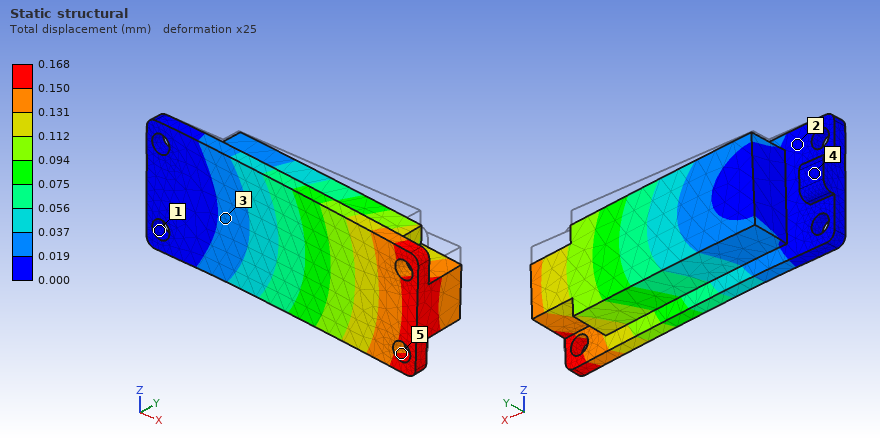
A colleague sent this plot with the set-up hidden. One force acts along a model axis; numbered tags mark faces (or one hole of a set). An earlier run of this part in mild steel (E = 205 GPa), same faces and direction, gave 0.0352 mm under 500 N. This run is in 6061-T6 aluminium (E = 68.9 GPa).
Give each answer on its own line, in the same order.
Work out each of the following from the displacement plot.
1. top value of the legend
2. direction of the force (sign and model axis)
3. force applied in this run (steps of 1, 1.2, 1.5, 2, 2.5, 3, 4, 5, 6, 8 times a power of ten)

0.168 mm
-Z
800 N
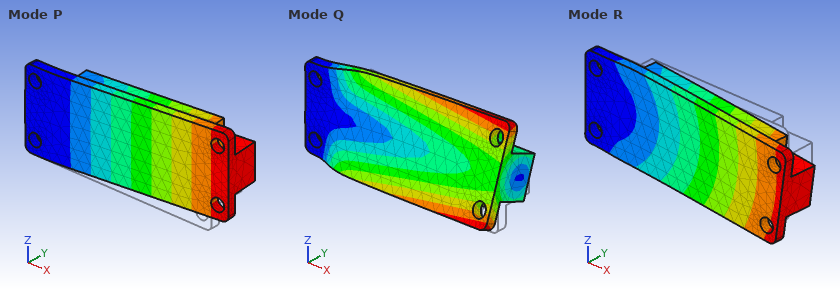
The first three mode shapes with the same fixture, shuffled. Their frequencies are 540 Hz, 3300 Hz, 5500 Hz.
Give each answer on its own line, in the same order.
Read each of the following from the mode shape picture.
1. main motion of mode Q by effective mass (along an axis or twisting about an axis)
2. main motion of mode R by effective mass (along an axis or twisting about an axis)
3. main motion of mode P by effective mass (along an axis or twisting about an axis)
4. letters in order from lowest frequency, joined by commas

twisting about X
along Z
along Y
P, R, Q
